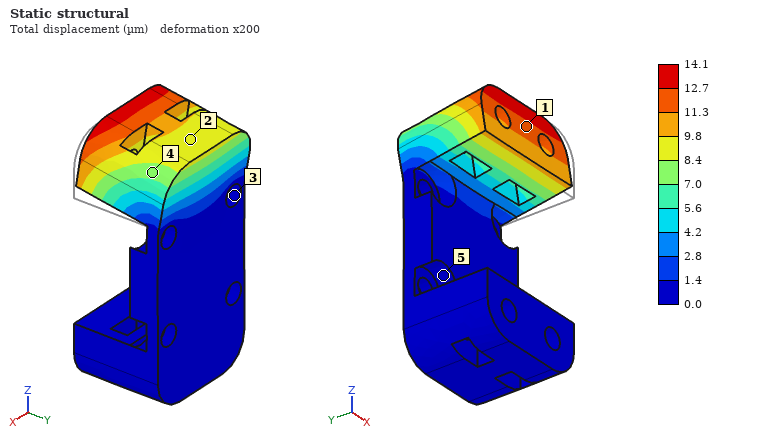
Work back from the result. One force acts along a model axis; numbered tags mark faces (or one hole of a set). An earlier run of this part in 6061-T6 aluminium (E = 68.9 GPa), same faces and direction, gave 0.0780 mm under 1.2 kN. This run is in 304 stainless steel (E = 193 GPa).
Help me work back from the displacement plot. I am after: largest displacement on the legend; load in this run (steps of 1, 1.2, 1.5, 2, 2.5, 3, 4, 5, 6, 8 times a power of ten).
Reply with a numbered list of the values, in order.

1. 14.1 µm
2. 600 N
